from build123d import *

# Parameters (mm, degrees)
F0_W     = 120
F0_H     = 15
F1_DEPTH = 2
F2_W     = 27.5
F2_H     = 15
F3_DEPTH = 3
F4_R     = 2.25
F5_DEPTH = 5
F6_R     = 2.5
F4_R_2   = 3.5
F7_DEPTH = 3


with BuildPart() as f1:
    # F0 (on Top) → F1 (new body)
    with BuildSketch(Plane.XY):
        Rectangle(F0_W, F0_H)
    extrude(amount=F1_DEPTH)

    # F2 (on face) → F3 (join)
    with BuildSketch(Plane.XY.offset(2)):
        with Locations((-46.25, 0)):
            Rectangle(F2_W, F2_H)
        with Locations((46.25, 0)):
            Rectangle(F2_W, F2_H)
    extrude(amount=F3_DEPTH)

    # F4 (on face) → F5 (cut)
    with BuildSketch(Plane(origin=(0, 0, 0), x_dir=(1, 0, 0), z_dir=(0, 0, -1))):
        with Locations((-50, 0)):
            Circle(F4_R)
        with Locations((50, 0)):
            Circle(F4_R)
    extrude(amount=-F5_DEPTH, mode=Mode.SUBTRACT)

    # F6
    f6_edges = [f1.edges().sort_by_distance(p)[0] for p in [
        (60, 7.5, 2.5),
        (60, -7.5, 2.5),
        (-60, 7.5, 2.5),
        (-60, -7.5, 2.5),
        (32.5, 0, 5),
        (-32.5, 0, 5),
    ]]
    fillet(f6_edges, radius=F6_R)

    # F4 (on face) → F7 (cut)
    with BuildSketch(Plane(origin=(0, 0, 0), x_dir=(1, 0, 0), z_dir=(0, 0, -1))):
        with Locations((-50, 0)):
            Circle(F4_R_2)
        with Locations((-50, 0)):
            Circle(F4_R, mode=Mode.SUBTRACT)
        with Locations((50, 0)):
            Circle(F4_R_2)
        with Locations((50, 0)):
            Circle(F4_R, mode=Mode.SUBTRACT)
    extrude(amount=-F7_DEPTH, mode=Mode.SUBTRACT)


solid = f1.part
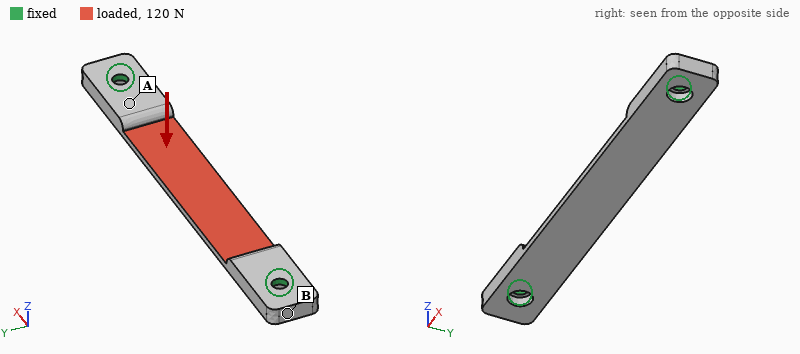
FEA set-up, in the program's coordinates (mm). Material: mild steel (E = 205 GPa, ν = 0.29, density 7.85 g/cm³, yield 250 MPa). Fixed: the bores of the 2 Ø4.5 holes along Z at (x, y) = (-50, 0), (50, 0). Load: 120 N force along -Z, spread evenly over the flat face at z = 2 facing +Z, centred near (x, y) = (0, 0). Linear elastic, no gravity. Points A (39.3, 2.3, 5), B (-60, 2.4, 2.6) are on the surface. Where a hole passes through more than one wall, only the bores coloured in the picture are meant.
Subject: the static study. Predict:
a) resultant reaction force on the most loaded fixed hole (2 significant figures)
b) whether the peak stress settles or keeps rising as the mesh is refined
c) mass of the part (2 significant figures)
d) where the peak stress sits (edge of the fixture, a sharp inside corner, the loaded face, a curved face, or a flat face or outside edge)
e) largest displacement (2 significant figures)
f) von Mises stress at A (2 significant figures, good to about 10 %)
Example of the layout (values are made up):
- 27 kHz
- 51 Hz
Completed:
- 220 N
- keeps rising
- 45 g
- edge of the fixture
- 65 µm
- 14 MPa
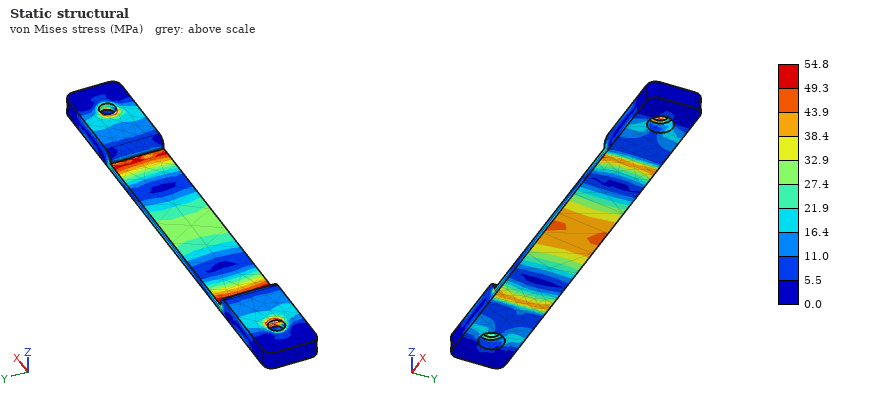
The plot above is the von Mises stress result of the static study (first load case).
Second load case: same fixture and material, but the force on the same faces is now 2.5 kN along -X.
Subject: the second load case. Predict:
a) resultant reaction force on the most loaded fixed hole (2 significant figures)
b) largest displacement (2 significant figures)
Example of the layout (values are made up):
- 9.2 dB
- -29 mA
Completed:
- 1.3 kN
- 34 µm
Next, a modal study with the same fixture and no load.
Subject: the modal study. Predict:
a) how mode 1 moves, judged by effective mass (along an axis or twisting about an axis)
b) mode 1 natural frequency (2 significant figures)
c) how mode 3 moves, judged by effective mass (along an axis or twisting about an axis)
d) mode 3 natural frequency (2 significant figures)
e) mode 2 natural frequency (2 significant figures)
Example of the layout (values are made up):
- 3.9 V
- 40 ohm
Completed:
- along Z
- 2000 Hz
- along Y
- 5900 Hz
- 4300 Hz
